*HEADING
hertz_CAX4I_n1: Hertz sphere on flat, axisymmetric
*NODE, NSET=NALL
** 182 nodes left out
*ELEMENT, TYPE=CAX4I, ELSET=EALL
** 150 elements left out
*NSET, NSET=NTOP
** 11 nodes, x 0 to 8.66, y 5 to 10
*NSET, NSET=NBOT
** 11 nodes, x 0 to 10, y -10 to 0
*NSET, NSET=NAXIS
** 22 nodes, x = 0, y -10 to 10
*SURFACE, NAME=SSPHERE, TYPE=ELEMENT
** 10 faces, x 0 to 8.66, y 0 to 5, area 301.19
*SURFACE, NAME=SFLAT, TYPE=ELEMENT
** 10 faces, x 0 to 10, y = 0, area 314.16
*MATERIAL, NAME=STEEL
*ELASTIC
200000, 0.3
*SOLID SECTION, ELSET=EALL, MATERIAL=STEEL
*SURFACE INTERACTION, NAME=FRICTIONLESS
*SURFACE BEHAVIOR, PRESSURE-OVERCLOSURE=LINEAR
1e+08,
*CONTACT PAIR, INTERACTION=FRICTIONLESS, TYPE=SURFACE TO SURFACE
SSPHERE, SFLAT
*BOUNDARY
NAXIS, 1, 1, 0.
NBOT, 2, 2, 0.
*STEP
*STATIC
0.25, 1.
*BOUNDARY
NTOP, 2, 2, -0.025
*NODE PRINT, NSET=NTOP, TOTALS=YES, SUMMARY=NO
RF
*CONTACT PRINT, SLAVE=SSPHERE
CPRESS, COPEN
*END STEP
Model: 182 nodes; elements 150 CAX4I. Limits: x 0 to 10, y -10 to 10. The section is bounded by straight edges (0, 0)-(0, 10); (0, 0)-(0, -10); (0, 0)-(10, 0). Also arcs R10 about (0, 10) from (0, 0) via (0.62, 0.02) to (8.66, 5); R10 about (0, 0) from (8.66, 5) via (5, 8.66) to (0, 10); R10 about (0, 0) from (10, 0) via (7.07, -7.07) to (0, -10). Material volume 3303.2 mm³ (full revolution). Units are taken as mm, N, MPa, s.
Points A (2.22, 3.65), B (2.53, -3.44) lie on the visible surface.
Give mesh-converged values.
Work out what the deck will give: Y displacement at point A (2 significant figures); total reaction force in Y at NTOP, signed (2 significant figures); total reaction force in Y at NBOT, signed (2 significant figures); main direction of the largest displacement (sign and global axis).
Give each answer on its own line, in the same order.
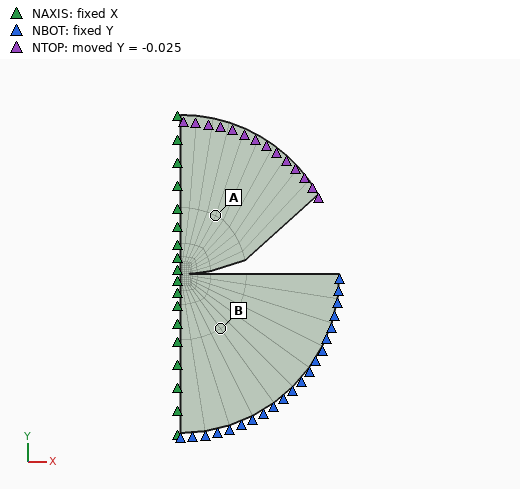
-0.024 mm
-1900 N
1900 N
-Y
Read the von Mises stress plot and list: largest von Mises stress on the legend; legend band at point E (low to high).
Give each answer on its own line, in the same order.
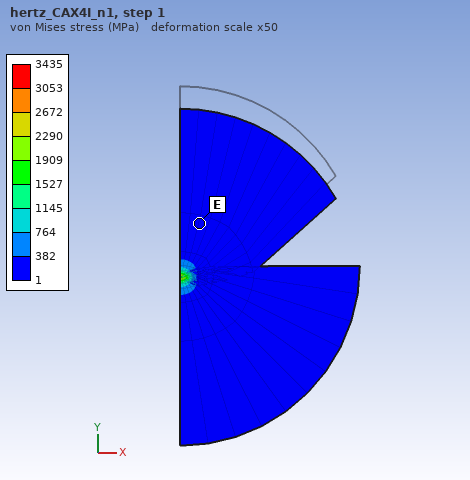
3435 MPa
1 to 382 MPa
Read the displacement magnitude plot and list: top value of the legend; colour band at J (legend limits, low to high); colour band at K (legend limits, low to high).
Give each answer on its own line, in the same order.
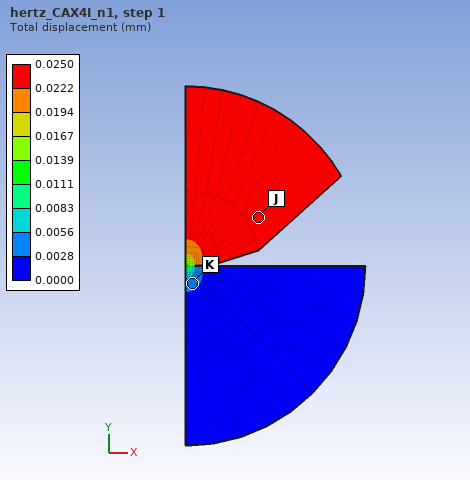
0.0250 mm
0.0222 to 0.0250 mm
0.0028 to 0.0056 mm
